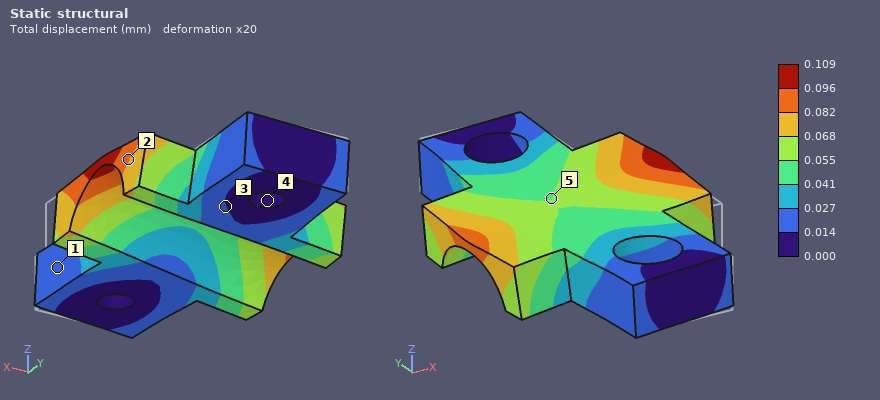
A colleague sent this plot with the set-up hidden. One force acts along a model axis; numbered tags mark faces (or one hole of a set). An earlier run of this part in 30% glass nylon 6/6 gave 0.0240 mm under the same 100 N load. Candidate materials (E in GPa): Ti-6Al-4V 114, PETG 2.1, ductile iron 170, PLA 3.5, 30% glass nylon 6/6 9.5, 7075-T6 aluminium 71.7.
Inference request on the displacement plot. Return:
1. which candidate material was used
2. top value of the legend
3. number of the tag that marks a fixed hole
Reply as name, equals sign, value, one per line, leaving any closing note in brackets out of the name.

which candidate material was used = PETG
top value of the legend = 0.109 mm
number of the tag that marks a fixed hole = 4
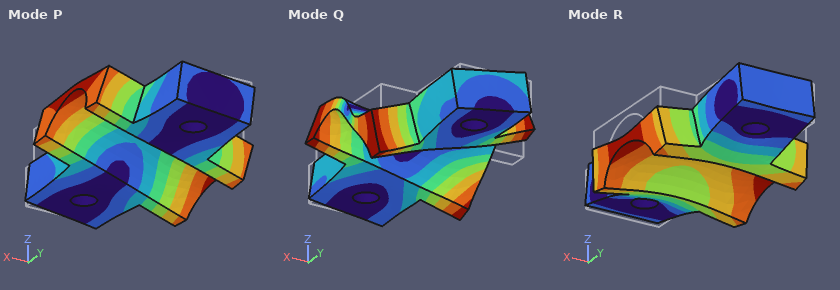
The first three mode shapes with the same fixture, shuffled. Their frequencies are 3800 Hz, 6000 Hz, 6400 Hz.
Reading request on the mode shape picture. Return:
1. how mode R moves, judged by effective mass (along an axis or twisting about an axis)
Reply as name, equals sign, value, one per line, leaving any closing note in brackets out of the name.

how mode R moves, judged by effective mass = along Z
